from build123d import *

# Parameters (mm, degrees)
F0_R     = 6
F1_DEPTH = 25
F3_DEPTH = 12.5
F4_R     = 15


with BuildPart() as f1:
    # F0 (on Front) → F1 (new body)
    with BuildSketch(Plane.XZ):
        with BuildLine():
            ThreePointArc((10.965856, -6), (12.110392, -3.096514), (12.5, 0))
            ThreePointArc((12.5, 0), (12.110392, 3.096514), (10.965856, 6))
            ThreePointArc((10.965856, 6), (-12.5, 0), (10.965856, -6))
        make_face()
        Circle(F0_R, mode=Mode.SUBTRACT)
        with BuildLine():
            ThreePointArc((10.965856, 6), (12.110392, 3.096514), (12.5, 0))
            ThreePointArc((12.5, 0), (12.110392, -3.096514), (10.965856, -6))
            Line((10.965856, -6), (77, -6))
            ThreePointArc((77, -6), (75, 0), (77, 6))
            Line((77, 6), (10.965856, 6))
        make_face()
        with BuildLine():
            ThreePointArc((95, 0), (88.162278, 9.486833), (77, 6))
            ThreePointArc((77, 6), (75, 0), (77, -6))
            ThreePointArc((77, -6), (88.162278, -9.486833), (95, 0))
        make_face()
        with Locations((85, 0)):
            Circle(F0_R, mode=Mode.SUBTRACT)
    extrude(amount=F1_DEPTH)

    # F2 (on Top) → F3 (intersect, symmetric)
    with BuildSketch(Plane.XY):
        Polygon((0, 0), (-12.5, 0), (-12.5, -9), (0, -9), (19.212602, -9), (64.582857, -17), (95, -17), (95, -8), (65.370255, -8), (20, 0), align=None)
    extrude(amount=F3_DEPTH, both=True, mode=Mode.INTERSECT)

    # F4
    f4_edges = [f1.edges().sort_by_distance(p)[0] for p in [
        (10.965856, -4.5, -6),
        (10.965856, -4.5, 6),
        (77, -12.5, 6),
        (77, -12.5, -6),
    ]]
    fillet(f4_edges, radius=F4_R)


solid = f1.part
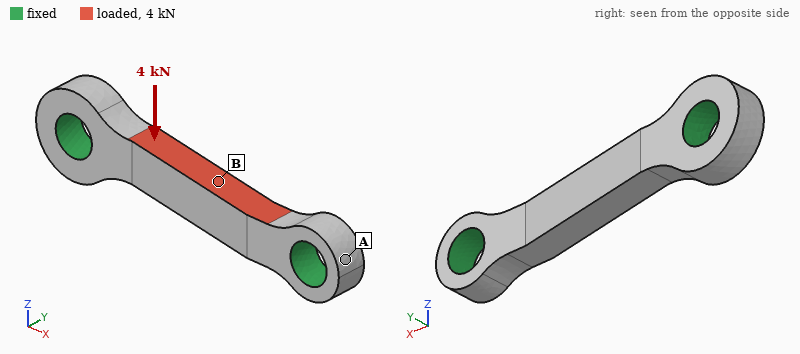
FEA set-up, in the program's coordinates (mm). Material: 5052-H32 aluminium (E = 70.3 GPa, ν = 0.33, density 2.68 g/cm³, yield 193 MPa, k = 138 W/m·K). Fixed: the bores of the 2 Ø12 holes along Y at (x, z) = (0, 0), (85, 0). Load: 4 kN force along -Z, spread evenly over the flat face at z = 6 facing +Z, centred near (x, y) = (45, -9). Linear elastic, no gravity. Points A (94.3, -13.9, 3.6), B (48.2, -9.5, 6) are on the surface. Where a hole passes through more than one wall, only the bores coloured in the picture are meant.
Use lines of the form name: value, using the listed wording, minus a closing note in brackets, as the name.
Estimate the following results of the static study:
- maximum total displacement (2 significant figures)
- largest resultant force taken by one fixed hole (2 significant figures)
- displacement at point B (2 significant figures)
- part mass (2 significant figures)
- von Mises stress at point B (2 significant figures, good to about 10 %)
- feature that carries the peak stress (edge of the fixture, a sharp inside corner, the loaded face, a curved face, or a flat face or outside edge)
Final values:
maximum total displacement: 71 µm
largest resultant force taken by one fixed hole: 2.1 kN
displacement at point B: 68 µm
part mass: 33 g
von Mises stress at point B: 66 MPa
feature that carries the peak stress: a curved face
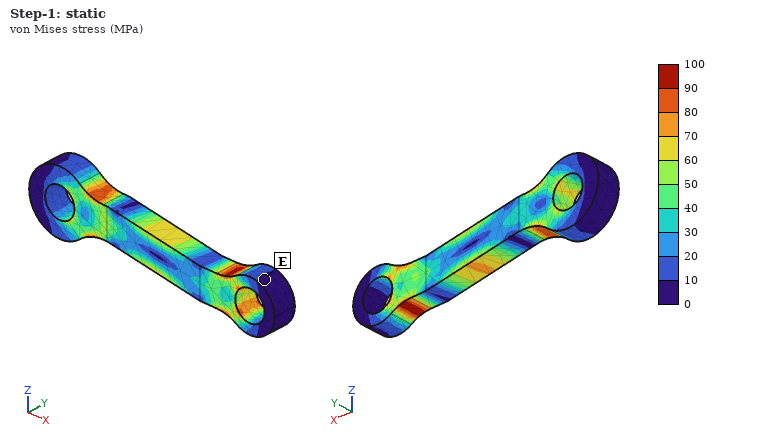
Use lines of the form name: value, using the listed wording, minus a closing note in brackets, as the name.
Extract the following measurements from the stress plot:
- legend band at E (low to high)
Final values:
legend band at E: 0 to 10 MPa
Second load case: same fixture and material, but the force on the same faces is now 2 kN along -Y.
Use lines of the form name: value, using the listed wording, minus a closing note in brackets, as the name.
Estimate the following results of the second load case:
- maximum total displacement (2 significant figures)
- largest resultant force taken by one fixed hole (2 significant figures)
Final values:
maximum total displacement: 81 µm
largest resultant force taken by one fixed hole: 1.1 kN
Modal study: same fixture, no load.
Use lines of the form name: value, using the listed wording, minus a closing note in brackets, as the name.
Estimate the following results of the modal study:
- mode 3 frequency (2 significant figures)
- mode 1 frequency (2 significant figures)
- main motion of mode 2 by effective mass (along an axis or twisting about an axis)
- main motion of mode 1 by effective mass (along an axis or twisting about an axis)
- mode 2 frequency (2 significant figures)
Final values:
mode 3 frequency: 20 kHz
mode 1 frequency: 8100 Hz
main motion of mode 2 by effective mass: along Z
main motion of mode 1 by effective mass: along Y
mode 2 frequency: 11 kHz
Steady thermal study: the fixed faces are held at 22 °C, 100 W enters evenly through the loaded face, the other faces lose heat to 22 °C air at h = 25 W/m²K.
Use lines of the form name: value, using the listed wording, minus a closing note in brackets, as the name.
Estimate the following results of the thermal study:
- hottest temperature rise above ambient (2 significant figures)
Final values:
hottest temperature rise above ambient: 80 K
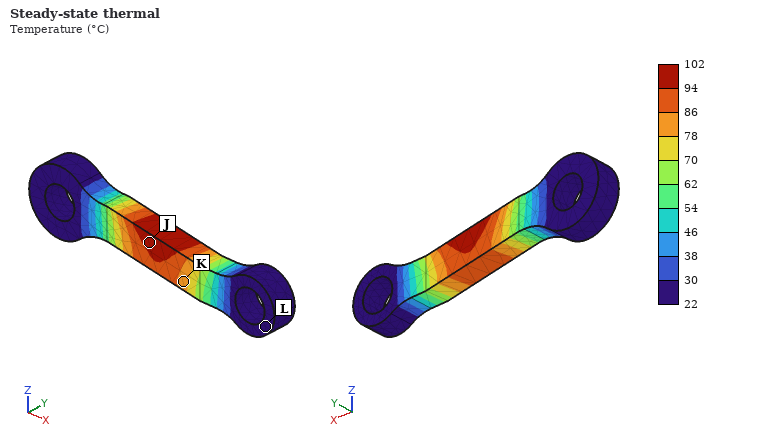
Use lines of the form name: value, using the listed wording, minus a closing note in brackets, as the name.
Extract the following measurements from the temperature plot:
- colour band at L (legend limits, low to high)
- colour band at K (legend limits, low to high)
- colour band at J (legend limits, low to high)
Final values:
colour band at L: 22 to 30 °C
colour band at K: 78 to 86 °C
colour band at J: 94 to 102 °C
